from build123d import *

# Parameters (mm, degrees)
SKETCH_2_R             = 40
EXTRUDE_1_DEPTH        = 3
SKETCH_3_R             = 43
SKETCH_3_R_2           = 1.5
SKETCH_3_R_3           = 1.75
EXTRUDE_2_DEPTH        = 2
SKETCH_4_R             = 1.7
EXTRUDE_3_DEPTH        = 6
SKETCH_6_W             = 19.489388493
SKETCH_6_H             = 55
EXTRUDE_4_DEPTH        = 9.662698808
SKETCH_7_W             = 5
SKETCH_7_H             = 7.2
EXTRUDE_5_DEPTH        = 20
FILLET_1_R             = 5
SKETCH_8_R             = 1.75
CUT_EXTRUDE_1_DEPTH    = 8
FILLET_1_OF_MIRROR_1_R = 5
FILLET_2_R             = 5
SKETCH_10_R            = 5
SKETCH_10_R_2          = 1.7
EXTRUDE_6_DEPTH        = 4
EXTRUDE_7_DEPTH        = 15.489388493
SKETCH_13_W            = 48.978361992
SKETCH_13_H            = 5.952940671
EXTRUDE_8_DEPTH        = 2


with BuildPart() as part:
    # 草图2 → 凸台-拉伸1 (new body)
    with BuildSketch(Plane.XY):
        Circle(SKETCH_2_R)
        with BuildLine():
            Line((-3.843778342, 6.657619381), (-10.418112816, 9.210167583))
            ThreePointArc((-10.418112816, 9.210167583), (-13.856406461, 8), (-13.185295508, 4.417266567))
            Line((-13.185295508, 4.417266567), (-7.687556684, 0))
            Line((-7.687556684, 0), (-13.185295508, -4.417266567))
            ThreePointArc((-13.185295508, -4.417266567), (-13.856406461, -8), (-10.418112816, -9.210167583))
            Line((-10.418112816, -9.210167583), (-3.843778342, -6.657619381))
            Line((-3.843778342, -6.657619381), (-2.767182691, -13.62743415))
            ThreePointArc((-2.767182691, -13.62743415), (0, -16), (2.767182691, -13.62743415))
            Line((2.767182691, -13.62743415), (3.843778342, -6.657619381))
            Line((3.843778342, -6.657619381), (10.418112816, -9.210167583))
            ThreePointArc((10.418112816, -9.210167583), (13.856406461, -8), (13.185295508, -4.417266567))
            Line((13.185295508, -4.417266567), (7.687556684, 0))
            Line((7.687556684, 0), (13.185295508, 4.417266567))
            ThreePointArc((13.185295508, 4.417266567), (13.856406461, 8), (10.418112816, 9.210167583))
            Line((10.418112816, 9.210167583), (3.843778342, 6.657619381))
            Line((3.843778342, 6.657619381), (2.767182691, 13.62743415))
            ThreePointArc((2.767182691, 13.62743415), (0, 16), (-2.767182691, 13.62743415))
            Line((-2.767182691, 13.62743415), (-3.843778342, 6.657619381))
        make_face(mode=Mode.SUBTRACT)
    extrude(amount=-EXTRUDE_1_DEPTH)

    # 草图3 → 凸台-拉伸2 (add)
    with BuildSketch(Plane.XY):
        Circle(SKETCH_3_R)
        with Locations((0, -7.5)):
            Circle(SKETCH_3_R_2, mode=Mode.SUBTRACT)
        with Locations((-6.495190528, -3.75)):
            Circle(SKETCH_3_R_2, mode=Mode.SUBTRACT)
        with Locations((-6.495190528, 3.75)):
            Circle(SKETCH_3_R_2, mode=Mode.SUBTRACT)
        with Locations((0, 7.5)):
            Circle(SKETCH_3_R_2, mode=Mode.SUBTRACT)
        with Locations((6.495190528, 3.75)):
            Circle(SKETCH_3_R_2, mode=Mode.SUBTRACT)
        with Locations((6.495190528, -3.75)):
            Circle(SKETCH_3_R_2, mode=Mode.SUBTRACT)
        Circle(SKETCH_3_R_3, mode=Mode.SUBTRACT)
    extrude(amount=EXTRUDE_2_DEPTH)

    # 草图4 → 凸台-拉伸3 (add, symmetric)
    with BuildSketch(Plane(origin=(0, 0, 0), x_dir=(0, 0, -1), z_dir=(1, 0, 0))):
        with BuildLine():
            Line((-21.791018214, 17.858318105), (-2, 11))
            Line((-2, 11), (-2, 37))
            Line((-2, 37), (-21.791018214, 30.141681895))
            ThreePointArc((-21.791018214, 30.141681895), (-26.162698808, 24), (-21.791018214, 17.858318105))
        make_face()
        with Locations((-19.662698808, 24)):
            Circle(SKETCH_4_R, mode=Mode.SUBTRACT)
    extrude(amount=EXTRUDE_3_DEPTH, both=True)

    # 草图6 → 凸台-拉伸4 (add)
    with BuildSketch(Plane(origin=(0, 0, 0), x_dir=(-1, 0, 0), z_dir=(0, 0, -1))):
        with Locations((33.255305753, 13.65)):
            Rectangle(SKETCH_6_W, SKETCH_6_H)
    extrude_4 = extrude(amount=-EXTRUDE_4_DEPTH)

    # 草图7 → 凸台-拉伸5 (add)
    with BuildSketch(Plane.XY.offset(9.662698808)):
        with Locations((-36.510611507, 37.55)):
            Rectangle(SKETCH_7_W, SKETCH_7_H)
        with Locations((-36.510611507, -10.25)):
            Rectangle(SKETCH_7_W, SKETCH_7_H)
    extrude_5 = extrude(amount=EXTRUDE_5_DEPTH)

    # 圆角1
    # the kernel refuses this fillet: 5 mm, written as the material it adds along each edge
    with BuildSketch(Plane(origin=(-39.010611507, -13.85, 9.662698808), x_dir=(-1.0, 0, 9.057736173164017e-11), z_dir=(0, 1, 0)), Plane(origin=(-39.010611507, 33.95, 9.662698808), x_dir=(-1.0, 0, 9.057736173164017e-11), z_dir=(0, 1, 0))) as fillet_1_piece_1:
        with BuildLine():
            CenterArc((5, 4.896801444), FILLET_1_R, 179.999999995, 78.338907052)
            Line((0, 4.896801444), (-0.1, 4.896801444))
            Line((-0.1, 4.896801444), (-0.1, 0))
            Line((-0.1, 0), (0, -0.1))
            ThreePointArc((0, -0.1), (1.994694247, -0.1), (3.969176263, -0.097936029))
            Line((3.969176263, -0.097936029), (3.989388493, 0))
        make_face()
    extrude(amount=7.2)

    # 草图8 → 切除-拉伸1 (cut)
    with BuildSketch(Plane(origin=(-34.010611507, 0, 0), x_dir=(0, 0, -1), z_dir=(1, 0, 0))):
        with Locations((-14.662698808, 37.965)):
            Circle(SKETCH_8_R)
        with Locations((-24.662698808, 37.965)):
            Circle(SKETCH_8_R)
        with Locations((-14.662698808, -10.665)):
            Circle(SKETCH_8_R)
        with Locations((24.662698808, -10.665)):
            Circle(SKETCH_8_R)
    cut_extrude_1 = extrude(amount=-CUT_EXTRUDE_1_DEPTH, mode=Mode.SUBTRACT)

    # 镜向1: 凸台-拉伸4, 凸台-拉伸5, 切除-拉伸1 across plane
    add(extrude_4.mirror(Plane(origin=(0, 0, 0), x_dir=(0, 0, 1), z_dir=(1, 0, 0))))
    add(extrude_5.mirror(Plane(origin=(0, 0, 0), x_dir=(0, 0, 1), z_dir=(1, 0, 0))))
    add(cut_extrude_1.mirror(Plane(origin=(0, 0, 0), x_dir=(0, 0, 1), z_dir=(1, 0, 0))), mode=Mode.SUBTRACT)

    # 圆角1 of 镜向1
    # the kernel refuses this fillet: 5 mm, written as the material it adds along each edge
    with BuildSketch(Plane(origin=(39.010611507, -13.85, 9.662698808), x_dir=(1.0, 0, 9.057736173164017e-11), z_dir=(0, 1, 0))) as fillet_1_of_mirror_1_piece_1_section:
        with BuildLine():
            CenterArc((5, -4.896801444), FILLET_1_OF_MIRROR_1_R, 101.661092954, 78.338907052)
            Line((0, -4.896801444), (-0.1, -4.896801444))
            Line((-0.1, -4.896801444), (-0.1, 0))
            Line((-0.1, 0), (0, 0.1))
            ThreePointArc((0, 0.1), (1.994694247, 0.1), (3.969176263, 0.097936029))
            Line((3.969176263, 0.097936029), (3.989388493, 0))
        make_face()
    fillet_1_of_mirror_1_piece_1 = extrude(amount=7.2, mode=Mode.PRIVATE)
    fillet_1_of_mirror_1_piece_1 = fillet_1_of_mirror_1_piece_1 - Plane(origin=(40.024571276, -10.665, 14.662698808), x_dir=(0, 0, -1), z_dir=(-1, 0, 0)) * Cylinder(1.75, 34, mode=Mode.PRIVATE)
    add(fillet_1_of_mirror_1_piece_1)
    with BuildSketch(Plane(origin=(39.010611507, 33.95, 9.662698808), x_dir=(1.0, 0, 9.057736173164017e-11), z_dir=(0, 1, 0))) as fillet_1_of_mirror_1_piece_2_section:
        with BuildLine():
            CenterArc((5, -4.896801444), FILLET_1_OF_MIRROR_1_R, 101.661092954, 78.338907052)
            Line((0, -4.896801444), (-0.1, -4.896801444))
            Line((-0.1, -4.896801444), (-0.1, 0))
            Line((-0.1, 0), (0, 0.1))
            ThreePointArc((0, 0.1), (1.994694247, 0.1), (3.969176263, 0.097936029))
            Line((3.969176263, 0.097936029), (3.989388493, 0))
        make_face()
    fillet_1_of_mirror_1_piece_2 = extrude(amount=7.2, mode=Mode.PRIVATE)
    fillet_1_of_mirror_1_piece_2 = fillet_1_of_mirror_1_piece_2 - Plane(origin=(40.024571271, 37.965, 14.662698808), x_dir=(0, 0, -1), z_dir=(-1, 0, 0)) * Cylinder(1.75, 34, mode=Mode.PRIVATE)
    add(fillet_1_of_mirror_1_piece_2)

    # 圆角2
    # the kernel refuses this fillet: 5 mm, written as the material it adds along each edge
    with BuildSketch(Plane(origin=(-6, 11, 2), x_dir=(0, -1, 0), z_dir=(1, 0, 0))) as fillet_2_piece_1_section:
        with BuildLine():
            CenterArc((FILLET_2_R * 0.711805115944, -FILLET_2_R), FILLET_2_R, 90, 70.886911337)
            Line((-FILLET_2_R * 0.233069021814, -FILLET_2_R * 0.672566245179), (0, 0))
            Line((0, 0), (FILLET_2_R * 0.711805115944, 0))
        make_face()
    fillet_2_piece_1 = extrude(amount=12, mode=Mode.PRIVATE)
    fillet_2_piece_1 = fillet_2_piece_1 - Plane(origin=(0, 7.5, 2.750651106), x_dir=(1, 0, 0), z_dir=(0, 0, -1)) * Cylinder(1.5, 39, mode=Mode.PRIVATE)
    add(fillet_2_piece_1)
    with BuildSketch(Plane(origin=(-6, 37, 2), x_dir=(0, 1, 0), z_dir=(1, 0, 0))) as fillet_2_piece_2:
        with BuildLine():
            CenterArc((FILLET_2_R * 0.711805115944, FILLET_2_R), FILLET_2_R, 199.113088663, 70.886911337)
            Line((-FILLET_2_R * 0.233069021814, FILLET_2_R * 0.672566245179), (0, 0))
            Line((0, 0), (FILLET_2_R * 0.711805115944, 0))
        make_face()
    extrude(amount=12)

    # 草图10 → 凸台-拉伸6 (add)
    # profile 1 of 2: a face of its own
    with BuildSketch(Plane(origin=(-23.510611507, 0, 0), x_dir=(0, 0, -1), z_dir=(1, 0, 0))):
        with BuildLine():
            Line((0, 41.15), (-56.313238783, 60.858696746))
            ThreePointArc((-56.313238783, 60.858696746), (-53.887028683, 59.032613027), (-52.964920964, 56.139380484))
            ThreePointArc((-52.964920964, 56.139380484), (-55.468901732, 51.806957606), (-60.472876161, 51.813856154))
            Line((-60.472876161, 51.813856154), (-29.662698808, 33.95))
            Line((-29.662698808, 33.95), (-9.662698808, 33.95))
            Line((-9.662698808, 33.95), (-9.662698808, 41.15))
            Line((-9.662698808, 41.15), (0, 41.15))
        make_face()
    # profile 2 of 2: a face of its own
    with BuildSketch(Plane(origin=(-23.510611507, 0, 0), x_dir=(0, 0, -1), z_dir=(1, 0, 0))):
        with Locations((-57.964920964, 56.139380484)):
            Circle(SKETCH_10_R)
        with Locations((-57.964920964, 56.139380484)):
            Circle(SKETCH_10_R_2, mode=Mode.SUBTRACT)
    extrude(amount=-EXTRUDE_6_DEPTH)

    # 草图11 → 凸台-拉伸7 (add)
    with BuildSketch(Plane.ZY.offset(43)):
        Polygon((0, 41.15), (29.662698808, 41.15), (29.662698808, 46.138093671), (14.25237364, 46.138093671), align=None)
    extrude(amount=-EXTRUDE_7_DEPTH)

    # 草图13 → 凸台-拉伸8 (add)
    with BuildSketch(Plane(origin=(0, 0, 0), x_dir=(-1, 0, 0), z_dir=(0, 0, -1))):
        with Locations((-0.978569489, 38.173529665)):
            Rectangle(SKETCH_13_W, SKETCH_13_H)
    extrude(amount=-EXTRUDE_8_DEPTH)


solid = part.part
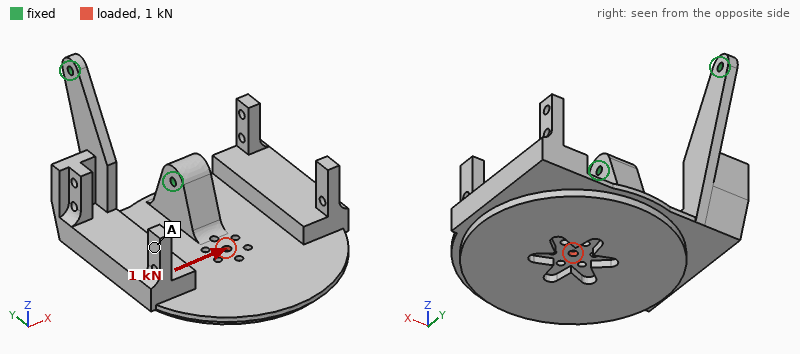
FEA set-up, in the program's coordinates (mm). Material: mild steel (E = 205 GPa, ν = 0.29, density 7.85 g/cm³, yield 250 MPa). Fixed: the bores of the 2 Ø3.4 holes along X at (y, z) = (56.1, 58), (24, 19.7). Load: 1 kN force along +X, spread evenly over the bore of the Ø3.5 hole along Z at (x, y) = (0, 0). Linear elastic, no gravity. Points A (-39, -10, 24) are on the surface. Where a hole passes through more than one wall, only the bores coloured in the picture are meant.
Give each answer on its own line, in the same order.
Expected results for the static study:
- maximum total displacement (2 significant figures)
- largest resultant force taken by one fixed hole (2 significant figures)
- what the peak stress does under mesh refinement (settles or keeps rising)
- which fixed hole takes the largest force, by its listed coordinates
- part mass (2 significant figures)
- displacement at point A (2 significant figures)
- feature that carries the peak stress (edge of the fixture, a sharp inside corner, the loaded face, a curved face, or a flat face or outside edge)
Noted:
54 µm
1.0 kN
keeps rising
(24, 19.7)
430 g
49 µm
edge of the fixture
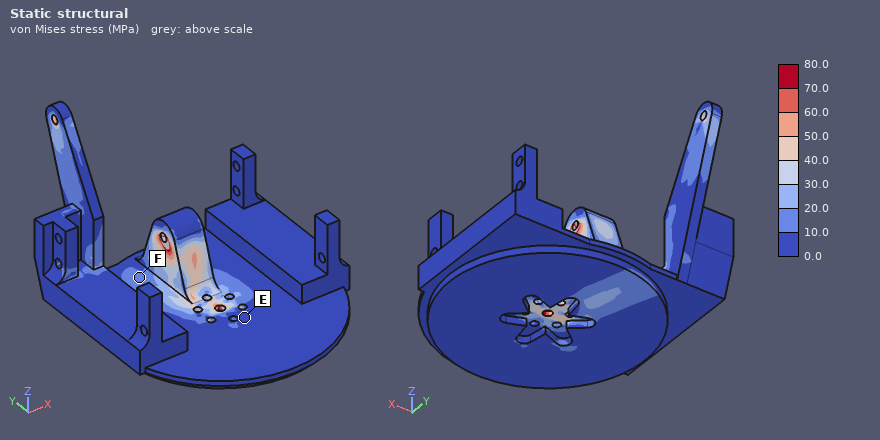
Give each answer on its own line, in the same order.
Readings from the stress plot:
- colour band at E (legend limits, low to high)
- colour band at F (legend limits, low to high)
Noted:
0.0 to 10.0 MPa
10.0 to 20.0 MPa
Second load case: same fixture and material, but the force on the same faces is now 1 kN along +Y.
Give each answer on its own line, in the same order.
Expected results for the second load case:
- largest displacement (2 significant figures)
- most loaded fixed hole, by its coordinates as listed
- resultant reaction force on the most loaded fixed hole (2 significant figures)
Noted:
30 µm
(24, 19.7)
960 N
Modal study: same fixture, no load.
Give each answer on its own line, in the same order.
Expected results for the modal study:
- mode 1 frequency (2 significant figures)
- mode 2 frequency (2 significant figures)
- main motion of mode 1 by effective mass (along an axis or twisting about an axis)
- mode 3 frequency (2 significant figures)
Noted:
1000 Hz
1100 Hz
along Z
1300 Hz
